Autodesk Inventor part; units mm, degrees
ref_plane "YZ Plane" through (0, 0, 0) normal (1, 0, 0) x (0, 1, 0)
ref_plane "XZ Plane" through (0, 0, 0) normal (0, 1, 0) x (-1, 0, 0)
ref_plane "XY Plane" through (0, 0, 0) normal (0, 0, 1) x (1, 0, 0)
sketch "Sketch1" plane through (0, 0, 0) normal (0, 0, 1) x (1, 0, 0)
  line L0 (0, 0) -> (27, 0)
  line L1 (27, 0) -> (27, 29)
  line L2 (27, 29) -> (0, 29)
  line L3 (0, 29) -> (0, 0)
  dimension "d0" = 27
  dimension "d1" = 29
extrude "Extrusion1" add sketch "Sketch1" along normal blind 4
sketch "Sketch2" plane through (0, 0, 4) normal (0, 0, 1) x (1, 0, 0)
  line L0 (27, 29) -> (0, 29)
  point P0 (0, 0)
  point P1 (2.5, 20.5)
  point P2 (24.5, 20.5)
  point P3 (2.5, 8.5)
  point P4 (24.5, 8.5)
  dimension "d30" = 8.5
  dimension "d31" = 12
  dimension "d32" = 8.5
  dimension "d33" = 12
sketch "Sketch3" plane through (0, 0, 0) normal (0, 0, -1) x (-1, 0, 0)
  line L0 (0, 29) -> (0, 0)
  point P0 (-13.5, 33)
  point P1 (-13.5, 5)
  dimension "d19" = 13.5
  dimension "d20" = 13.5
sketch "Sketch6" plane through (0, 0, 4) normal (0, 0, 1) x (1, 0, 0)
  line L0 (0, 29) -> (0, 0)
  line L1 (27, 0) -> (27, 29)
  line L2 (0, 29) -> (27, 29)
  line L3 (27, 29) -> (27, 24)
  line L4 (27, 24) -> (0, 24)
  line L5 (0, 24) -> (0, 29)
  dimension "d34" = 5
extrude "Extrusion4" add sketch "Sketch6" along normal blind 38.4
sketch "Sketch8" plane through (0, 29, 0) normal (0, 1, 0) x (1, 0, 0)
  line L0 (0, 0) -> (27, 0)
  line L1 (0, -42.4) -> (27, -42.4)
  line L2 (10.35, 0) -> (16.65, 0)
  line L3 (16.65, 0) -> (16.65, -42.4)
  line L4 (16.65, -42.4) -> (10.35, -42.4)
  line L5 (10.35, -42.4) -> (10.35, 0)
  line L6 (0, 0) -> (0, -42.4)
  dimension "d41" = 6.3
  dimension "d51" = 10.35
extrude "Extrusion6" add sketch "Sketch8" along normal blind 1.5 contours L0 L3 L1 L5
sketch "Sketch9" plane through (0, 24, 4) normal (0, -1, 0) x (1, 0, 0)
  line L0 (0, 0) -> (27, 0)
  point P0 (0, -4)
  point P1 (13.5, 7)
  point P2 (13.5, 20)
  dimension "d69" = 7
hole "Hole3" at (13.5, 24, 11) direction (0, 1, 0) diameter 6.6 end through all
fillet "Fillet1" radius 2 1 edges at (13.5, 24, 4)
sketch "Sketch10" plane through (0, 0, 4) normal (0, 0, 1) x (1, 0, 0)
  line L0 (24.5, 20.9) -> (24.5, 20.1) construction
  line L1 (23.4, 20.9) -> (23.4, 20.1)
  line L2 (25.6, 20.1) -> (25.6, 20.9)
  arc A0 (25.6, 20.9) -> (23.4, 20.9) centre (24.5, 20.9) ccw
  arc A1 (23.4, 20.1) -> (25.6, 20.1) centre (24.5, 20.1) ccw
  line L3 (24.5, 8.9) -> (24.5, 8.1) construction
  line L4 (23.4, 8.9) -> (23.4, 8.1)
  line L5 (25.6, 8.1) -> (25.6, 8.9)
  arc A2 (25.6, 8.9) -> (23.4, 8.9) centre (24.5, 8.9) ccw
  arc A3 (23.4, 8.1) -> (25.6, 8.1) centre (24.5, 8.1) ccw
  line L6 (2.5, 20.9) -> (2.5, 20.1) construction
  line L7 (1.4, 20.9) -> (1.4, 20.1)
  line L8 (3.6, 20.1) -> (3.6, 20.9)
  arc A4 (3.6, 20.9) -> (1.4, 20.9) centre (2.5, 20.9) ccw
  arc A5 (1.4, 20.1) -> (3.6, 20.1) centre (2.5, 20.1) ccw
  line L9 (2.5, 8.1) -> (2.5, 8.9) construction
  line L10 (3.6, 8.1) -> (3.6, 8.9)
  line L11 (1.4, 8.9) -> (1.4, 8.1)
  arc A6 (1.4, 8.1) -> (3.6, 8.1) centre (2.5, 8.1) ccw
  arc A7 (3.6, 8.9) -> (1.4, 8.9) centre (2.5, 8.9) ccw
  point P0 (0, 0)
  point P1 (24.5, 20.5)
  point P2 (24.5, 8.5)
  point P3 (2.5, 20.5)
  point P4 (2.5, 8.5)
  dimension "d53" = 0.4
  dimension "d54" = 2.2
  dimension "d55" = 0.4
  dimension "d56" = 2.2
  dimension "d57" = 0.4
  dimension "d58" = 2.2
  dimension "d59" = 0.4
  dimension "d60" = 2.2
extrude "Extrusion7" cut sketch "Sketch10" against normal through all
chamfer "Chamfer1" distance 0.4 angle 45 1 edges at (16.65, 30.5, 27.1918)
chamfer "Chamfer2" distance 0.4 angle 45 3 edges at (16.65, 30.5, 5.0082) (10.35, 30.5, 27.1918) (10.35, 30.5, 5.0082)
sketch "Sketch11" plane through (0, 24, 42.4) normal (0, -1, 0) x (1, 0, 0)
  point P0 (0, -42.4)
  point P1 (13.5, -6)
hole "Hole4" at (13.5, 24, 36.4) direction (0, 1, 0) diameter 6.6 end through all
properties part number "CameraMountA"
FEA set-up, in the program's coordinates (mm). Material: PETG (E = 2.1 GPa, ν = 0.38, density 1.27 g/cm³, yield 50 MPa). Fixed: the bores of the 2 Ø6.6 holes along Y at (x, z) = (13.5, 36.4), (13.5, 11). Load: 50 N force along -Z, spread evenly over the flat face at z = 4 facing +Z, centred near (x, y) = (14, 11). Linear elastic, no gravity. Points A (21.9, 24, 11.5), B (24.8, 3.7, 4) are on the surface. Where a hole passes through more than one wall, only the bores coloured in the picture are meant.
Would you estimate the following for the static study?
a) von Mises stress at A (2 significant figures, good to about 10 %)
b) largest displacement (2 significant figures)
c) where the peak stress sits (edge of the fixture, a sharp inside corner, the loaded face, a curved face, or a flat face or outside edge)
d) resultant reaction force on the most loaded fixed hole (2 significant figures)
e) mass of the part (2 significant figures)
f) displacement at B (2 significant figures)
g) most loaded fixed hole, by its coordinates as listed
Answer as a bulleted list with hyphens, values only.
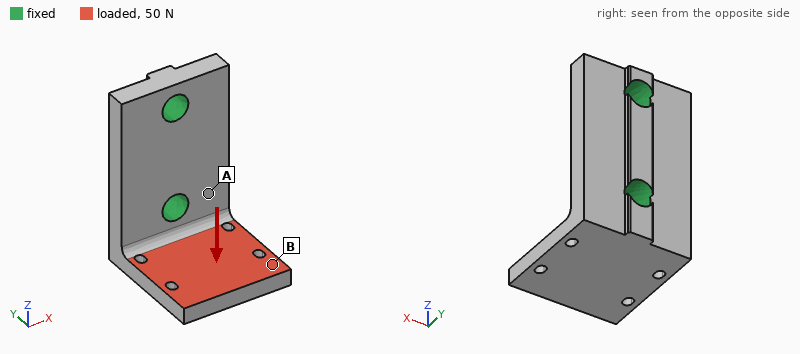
- 2.1 MPa
- 0.54 mm
- a sharp inside corner
- 44 N
- 10 g
- 0.44 mm
- (13.5, 11)
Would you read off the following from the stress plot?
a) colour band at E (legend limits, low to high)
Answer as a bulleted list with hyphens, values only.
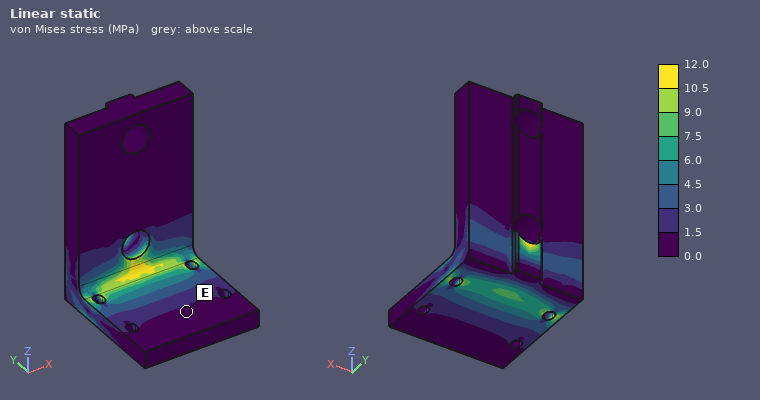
- 0.0 to 1.5 MPa
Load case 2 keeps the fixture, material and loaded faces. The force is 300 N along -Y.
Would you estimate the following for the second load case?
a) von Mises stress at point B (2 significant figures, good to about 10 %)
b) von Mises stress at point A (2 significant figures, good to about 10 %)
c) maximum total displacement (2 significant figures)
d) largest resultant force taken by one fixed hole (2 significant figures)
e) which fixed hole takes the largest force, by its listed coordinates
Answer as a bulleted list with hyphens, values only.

- 1.9 MPa
- 3.4 MPa
- 0.29 mm
- 310 N
- (13.5, 11)
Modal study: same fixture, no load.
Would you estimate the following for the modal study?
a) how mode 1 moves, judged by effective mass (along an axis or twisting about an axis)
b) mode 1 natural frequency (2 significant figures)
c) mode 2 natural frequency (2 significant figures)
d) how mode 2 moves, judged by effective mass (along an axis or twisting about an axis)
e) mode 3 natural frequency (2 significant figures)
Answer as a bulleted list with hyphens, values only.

- along Z
- 1100 Hz
- 1800 Hz
- along X
- 2600 Hz
